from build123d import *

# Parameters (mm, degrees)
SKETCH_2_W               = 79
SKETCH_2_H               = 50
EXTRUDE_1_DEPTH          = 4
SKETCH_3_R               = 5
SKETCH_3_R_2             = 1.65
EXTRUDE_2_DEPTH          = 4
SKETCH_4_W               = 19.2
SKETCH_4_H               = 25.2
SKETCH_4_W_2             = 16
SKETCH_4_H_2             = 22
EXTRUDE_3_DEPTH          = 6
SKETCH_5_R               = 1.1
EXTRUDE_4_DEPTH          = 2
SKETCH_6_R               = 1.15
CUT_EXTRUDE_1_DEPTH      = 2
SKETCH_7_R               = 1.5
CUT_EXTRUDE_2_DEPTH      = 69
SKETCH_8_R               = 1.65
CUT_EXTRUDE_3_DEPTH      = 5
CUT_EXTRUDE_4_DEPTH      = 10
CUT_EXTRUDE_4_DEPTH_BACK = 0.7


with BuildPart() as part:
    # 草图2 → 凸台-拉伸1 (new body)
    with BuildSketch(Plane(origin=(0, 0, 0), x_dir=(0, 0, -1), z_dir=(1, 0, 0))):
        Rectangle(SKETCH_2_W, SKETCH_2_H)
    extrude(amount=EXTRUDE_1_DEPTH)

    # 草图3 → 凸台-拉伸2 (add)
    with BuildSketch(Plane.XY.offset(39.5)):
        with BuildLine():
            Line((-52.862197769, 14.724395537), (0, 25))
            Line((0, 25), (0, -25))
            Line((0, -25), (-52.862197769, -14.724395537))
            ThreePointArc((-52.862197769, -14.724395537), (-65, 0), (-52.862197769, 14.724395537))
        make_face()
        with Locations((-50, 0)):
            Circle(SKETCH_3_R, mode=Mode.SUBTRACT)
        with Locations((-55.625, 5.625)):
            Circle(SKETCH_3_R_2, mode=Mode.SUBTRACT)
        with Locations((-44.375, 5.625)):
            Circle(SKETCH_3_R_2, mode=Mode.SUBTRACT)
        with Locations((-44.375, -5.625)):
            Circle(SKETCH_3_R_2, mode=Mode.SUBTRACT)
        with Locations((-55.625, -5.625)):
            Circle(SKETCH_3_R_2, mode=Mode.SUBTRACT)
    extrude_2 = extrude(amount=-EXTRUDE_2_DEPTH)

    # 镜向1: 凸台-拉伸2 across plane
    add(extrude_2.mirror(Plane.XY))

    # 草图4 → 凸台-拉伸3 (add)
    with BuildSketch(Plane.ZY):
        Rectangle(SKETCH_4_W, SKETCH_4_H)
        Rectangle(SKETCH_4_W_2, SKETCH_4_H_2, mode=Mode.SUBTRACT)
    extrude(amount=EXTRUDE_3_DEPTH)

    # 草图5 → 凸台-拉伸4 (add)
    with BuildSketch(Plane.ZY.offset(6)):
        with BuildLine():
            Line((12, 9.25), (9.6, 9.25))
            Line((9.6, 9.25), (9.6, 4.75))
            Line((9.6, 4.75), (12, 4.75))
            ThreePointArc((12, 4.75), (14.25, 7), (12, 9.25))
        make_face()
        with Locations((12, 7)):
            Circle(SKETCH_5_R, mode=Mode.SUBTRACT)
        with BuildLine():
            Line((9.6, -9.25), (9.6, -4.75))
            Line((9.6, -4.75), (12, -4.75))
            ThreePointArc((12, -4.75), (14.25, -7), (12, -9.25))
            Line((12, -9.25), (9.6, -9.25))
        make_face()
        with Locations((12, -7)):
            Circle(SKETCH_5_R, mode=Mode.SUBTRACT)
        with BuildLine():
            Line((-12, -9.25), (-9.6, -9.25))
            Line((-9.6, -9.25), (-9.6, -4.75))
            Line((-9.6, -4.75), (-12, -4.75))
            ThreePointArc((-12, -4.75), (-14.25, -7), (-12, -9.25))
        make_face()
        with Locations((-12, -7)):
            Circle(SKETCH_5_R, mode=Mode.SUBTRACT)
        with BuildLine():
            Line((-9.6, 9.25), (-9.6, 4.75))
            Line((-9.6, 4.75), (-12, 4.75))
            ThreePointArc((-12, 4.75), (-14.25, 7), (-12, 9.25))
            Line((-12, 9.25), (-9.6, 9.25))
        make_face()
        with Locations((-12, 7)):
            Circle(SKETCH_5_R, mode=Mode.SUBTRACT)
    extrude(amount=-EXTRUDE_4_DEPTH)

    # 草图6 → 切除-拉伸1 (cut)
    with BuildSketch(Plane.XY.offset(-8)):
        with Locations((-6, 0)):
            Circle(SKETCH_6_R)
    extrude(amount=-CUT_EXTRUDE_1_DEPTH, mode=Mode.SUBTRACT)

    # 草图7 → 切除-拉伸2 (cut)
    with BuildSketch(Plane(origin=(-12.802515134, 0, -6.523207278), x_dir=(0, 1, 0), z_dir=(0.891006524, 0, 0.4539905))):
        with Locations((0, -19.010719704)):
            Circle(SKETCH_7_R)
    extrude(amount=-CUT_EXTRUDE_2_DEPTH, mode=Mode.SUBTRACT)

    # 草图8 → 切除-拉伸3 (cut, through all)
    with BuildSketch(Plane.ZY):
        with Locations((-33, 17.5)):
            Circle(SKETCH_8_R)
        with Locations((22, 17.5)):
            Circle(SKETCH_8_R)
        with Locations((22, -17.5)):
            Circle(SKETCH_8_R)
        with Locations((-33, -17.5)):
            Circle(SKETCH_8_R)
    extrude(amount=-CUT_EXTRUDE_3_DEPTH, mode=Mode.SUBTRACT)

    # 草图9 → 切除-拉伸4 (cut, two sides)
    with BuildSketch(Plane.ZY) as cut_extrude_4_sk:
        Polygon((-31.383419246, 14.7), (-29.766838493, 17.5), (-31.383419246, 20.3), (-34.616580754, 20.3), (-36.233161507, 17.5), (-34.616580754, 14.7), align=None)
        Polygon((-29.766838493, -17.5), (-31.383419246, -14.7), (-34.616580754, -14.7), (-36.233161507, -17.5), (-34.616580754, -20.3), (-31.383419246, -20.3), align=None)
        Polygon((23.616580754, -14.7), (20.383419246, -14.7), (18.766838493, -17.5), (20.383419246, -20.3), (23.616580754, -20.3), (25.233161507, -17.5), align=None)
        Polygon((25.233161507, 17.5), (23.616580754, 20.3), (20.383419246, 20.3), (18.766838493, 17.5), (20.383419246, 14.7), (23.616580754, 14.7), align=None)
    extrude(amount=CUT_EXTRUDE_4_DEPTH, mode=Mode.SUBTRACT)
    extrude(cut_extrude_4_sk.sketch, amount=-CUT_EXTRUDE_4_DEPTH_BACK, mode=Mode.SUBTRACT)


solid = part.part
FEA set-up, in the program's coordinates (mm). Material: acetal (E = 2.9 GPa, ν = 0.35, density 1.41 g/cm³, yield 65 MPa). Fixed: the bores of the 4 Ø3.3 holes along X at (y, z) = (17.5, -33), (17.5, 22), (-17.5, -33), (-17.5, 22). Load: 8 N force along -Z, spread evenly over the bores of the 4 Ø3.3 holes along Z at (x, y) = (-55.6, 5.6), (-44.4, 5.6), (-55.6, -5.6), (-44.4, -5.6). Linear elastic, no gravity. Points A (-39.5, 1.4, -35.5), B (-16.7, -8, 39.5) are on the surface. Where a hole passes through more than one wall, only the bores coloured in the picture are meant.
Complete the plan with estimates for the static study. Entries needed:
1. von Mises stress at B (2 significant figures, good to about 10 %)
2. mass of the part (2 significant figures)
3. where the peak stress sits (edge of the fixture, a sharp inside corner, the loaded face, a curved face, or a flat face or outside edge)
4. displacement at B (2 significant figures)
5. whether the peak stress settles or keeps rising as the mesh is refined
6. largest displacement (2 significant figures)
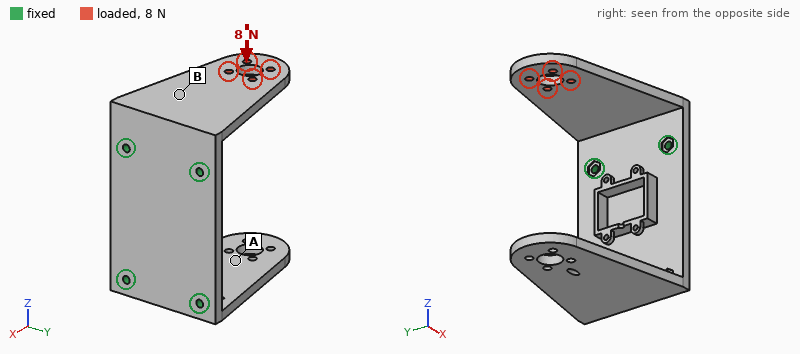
2.1 MPa
49 g
edge of the fixture
0.27 mm
keeps rising
1.3 mm
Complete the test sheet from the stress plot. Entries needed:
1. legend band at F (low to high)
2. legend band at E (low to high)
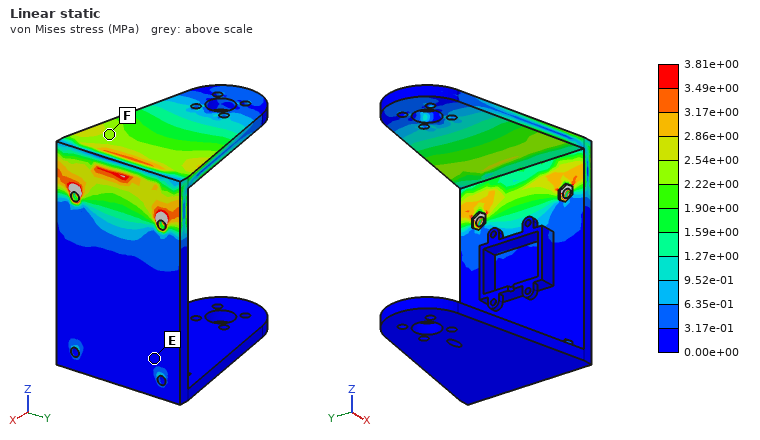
2.22e+00 to 2.54e+00 MPa
0.00e+00 to 3.17e-01 MPa
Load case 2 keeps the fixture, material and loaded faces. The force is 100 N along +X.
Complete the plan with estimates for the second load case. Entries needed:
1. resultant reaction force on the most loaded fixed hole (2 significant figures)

55 N
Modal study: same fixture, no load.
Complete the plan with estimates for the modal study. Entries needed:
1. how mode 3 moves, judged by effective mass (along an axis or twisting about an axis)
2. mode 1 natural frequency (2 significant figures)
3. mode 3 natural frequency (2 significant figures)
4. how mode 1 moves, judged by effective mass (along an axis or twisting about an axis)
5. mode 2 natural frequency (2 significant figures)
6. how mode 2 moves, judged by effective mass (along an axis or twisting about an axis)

along Y
210 Hz
600 Hz
along Z
250 Hz
along Z
